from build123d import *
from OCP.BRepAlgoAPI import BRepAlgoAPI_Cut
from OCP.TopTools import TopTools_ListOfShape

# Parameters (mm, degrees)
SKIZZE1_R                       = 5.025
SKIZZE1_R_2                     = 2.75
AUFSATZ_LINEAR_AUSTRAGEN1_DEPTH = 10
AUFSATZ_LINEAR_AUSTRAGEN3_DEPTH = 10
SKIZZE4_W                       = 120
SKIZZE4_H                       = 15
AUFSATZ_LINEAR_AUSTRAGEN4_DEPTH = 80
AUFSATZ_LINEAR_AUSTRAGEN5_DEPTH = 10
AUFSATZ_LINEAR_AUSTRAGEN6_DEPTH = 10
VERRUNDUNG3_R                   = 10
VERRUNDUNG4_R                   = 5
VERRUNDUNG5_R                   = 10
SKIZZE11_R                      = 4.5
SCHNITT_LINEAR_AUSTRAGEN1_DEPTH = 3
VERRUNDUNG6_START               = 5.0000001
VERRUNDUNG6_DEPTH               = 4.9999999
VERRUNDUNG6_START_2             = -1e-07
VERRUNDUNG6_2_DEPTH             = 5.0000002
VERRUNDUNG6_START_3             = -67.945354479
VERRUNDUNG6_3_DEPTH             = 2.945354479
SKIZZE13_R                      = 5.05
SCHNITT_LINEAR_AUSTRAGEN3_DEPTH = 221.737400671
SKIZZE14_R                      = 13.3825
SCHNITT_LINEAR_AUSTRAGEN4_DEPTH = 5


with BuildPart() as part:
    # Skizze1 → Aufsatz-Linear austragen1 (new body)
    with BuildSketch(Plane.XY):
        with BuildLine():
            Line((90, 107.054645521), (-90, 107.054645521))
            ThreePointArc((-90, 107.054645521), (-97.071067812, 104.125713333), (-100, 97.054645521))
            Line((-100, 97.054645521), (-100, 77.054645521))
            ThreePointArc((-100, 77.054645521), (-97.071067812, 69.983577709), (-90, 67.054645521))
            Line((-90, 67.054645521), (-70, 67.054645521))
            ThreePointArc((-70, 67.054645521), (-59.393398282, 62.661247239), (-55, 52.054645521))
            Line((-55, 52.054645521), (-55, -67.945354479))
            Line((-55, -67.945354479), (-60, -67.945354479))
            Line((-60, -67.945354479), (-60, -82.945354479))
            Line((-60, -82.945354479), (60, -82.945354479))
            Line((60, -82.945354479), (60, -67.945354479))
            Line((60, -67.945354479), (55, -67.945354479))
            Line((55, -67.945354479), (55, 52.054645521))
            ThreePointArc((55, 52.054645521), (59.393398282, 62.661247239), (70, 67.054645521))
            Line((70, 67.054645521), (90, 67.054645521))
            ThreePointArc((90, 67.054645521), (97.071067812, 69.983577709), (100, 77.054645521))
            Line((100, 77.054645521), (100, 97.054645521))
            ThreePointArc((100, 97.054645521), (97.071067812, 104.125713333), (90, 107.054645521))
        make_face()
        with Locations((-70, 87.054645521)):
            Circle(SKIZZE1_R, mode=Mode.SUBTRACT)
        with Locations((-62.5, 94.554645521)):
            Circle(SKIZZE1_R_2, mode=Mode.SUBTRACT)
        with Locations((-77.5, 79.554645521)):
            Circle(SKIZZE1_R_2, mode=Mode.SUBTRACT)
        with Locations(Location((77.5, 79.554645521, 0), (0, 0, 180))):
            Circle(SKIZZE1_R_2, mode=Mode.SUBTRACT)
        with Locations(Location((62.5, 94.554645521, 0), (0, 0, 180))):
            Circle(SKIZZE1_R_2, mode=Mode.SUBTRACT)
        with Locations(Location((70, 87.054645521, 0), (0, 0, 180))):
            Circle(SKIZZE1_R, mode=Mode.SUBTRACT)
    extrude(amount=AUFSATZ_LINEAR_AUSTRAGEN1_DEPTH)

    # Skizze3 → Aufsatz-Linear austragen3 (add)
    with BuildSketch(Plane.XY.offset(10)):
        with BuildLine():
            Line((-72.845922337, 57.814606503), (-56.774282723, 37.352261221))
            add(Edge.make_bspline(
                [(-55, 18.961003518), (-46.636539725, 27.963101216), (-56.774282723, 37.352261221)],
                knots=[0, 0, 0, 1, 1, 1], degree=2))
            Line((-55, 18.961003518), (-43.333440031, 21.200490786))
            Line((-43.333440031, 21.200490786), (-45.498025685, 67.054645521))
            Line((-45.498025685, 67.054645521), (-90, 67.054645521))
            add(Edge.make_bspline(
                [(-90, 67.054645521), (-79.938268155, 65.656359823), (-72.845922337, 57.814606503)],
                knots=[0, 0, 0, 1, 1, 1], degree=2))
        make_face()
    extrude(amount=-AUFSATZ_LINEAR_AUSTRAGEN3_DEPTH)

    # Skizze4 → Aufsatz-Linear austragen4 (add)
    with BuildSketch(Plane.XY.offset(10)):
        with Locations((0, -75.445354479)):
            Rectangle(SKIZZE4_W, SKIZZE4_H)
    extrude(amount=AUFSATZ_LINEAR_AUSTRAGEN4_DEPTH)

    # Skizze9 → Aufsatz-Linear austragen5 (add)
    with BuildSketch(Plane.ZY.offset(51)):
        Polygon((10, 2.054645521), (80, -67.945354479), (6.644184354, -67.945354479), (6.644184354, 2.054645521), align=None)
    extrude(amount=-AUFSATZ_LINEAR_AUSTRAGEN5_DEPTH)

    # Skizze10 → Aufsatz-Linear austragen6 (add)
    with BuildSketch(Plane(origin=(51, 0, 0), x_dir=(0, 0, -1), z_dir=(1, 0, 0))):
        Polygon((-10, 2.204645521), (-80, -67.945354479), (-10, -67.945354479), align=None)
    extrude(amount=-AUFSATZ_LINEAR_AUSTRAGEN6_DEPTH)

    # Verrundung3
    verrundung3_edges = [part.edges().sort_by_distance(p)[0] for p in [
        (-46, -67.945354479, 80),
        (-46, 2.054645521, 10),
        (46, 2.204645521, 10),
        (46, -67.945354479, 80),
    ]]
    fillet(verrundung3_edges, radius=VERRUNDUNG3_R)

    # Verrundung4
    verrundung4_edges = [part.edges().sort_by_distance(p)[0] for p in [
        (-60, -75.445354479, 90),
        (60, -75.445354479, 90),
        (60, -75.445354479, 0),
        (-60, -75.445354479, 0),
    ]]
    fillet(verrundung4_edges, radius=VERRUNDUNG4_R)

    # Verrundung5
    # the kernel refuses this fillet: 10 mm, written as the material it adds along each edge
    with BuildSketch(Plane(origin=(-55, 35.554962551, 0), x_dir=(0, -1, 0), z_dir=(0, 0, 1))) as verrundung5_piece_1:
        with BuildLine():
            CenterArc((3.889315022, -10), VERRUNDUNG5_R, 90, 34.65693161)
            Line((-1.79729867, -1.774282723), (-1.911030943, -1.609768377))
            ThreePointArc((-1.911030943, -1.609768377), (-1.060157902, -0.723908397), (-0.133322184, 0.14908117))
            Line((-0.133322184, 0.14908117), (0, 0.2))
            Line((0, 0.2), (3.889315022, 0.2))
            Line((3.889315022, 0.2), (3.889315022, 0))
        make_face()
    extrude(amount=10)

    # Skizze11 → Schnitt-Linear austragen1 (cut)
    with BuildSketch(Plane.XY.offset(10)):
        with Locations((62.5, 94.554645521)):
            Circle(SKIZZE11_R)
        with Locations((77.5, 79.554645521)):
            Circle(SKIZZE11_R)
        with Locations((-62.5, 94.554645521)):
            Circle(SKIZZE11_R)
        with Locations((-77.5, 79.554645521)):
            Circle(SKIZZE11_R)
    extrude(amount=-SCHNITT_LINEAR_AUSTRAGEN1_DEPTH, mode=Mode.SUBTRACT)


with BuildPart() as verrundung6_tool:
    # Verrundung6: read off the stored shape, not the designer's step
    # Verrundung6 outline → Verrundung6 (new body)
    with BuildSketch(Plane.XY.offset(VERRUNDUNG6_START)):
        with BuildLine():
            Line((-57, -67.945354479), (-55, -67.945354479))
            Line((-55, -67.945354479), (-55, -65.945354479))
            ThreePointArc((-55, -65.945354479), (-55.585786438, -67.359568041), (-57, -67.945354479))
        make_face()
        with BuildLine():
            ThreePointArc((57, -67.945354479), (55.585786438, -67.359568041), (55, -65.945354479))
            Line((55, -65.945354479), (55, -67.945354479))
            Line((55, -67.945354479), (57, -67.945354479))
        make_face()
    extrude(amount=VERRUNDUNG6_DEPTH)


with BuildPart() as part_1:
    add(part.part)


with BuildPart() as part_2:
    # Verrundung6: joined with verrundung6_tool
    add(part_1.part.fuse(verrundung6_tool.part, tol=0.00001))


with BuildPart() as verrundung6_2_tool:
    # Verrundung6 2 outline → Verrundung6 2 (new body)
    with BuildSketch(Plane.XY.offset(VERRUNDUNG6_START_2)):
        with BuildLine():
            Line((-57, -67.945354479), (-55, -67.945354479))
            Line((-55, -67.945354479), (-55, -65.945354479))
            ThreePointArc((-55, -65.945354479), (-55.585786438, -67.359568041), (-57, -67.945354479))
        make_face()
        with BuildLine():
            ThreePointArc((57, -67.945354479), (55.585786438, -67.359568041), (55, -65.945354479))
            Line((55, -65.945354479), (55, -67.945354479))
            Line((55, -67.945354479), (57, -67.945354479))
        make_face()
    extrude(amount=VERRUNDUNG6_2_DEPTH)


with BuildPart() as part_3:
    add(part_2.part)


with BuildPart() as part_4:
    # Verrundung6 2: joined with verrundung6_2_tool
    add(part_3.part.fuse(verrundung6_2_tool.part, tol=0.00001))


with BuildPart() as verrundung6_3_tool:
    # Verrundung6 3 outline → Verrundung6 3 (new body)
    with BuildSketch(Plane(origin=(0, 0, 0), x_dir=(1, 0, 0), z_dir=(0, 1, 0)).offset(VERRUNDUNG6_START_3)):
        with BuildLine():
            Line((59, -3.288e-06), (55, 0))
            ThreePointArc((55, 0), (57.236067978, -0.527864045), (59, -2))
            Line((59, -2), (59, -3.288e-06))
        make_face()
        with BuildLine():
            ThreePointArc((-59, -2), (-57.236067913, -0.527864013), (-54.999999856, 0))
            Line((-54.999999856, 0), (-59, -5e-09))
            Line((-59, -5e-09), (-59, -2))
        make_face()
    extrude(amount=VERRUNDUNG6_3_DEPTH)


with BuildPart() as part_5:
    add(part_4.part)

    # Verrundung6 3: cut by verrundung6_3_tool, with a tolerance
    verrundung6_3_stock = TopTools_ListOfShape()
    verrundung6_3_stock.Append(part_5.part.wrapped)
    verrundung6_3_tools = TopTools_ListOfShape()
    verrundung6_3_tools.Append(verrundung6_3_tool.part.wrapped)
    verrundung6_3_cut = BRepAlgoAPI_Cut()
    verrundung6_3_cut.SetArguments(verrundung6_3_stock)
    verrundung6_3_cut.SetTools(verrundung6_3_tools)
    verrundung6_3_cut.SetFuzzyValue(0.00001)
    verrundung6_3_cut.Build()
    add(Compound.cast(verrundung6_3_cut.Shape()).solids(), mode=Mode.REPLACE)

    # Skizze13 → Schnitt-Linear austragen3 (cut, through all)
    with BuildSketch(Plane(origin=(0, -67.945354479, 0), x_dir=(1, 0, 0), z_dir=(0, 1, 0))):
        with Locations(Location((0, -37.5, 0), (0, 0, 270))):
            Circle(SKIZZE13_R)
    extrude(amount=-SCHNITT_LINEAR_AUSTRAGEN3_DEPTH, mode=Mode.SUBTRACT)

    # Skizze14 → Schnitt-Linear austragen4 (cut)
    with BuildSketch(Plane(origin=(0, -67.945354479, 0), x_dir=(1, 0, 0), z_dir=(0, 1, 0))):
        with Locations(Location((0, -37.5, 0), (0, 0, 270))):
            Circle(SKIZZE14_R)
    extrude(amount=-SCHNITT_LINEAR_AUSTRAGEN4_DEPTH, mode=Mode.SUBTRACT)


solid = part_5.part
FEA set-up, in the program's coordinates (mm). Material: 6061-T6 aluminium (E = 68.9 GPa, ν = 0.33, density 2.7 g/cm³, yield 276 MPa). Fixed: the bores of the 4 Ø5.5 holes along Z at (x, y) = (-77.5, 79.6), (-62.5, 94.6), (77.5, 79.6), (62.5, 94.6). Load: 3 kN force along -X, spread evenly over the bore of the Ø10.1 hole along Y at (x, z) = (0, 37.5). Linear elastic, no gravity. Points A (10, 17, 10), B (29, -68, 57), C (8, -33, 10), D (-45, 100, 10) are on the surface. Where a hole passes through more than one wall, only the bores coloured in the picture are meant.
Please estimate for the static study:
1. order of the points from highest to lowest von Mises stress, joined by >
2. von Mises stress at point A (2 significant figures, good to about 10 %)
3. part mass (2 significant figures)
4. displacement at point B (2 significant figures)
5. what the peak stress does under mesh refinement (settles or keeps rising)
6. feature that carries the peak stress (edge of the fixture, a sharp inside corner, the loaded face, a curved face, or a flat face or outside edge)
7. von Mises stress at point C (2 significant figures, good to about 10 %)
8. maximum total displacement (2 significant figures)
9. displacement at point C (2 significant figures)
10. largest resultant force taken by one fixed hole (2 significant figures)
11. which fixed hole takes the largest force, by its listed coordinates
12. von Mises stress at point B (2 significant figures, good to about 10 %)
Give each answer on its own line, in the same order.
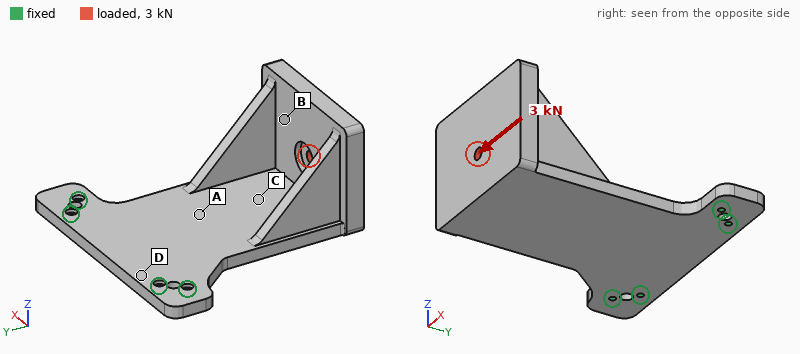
A > C > B > D
31 MPa
1.2 kg
0.47 mm
keeps rising
edge of the fixture
16 MPa
0.75 mm
0.12 mm
3.0 kN
(62.5, 94.6)
12 MPa
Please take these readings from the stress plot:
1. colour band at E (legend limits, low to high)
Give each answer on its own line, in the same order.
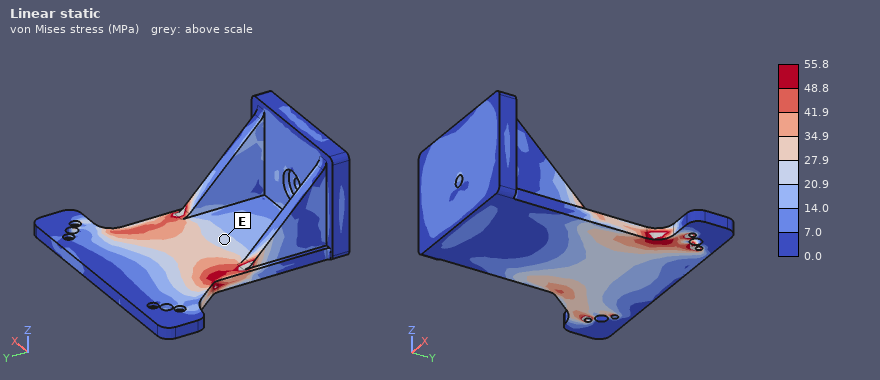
20.9 to 27.9 MPa
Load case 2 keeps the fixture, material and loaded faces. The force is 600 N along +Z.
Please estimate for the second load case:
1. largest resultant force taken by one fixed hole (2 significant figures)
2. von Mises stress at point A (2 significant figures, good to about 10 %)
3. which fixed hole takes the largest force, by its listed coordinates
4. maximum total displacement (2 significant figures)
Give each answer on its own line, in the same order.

1.4 kN
29 MPa
(-77.5, 79.6)
2.1 mm
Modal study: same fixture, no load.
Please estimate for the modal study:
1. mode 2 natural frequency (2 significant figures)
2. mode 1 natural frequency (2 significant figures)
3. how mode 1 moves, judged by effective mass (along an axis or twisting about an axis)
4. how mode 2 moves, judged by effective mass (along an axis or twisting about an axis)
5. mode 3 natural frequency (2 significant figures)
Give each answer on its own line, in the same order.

420 Hz
120 Hz
along Z
along X
870 Hz
